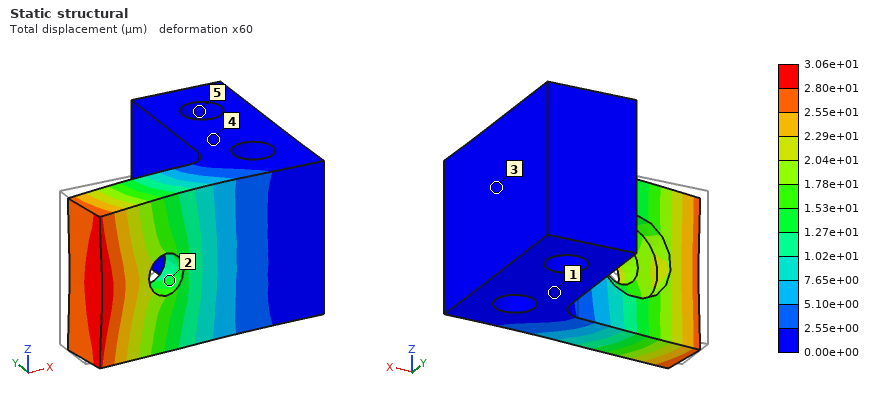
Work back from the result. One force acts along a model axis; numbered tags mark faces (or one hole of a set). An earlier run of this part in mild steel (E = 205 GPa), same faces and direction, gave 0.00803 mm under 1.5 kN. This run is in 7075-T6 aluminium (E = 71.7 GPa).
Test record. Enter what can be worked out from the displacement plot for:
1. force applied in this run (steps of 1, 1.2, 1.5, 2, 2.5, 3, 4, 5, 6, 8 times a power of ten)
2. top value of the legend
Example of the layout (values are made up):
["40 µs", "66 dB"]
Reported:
["2 kN", "3.06e+01 µm"]
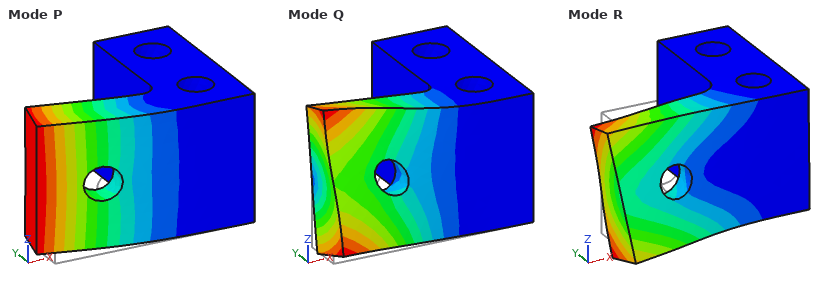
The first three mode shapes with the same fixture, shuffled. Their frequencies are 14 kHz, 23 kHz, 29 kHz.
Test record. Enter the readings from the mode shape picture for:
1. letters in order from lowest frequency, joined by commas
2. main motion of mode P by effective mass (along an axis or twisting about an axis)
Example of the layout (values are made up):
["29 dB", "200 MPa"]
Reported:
["P, R, Q", "along Y"]
